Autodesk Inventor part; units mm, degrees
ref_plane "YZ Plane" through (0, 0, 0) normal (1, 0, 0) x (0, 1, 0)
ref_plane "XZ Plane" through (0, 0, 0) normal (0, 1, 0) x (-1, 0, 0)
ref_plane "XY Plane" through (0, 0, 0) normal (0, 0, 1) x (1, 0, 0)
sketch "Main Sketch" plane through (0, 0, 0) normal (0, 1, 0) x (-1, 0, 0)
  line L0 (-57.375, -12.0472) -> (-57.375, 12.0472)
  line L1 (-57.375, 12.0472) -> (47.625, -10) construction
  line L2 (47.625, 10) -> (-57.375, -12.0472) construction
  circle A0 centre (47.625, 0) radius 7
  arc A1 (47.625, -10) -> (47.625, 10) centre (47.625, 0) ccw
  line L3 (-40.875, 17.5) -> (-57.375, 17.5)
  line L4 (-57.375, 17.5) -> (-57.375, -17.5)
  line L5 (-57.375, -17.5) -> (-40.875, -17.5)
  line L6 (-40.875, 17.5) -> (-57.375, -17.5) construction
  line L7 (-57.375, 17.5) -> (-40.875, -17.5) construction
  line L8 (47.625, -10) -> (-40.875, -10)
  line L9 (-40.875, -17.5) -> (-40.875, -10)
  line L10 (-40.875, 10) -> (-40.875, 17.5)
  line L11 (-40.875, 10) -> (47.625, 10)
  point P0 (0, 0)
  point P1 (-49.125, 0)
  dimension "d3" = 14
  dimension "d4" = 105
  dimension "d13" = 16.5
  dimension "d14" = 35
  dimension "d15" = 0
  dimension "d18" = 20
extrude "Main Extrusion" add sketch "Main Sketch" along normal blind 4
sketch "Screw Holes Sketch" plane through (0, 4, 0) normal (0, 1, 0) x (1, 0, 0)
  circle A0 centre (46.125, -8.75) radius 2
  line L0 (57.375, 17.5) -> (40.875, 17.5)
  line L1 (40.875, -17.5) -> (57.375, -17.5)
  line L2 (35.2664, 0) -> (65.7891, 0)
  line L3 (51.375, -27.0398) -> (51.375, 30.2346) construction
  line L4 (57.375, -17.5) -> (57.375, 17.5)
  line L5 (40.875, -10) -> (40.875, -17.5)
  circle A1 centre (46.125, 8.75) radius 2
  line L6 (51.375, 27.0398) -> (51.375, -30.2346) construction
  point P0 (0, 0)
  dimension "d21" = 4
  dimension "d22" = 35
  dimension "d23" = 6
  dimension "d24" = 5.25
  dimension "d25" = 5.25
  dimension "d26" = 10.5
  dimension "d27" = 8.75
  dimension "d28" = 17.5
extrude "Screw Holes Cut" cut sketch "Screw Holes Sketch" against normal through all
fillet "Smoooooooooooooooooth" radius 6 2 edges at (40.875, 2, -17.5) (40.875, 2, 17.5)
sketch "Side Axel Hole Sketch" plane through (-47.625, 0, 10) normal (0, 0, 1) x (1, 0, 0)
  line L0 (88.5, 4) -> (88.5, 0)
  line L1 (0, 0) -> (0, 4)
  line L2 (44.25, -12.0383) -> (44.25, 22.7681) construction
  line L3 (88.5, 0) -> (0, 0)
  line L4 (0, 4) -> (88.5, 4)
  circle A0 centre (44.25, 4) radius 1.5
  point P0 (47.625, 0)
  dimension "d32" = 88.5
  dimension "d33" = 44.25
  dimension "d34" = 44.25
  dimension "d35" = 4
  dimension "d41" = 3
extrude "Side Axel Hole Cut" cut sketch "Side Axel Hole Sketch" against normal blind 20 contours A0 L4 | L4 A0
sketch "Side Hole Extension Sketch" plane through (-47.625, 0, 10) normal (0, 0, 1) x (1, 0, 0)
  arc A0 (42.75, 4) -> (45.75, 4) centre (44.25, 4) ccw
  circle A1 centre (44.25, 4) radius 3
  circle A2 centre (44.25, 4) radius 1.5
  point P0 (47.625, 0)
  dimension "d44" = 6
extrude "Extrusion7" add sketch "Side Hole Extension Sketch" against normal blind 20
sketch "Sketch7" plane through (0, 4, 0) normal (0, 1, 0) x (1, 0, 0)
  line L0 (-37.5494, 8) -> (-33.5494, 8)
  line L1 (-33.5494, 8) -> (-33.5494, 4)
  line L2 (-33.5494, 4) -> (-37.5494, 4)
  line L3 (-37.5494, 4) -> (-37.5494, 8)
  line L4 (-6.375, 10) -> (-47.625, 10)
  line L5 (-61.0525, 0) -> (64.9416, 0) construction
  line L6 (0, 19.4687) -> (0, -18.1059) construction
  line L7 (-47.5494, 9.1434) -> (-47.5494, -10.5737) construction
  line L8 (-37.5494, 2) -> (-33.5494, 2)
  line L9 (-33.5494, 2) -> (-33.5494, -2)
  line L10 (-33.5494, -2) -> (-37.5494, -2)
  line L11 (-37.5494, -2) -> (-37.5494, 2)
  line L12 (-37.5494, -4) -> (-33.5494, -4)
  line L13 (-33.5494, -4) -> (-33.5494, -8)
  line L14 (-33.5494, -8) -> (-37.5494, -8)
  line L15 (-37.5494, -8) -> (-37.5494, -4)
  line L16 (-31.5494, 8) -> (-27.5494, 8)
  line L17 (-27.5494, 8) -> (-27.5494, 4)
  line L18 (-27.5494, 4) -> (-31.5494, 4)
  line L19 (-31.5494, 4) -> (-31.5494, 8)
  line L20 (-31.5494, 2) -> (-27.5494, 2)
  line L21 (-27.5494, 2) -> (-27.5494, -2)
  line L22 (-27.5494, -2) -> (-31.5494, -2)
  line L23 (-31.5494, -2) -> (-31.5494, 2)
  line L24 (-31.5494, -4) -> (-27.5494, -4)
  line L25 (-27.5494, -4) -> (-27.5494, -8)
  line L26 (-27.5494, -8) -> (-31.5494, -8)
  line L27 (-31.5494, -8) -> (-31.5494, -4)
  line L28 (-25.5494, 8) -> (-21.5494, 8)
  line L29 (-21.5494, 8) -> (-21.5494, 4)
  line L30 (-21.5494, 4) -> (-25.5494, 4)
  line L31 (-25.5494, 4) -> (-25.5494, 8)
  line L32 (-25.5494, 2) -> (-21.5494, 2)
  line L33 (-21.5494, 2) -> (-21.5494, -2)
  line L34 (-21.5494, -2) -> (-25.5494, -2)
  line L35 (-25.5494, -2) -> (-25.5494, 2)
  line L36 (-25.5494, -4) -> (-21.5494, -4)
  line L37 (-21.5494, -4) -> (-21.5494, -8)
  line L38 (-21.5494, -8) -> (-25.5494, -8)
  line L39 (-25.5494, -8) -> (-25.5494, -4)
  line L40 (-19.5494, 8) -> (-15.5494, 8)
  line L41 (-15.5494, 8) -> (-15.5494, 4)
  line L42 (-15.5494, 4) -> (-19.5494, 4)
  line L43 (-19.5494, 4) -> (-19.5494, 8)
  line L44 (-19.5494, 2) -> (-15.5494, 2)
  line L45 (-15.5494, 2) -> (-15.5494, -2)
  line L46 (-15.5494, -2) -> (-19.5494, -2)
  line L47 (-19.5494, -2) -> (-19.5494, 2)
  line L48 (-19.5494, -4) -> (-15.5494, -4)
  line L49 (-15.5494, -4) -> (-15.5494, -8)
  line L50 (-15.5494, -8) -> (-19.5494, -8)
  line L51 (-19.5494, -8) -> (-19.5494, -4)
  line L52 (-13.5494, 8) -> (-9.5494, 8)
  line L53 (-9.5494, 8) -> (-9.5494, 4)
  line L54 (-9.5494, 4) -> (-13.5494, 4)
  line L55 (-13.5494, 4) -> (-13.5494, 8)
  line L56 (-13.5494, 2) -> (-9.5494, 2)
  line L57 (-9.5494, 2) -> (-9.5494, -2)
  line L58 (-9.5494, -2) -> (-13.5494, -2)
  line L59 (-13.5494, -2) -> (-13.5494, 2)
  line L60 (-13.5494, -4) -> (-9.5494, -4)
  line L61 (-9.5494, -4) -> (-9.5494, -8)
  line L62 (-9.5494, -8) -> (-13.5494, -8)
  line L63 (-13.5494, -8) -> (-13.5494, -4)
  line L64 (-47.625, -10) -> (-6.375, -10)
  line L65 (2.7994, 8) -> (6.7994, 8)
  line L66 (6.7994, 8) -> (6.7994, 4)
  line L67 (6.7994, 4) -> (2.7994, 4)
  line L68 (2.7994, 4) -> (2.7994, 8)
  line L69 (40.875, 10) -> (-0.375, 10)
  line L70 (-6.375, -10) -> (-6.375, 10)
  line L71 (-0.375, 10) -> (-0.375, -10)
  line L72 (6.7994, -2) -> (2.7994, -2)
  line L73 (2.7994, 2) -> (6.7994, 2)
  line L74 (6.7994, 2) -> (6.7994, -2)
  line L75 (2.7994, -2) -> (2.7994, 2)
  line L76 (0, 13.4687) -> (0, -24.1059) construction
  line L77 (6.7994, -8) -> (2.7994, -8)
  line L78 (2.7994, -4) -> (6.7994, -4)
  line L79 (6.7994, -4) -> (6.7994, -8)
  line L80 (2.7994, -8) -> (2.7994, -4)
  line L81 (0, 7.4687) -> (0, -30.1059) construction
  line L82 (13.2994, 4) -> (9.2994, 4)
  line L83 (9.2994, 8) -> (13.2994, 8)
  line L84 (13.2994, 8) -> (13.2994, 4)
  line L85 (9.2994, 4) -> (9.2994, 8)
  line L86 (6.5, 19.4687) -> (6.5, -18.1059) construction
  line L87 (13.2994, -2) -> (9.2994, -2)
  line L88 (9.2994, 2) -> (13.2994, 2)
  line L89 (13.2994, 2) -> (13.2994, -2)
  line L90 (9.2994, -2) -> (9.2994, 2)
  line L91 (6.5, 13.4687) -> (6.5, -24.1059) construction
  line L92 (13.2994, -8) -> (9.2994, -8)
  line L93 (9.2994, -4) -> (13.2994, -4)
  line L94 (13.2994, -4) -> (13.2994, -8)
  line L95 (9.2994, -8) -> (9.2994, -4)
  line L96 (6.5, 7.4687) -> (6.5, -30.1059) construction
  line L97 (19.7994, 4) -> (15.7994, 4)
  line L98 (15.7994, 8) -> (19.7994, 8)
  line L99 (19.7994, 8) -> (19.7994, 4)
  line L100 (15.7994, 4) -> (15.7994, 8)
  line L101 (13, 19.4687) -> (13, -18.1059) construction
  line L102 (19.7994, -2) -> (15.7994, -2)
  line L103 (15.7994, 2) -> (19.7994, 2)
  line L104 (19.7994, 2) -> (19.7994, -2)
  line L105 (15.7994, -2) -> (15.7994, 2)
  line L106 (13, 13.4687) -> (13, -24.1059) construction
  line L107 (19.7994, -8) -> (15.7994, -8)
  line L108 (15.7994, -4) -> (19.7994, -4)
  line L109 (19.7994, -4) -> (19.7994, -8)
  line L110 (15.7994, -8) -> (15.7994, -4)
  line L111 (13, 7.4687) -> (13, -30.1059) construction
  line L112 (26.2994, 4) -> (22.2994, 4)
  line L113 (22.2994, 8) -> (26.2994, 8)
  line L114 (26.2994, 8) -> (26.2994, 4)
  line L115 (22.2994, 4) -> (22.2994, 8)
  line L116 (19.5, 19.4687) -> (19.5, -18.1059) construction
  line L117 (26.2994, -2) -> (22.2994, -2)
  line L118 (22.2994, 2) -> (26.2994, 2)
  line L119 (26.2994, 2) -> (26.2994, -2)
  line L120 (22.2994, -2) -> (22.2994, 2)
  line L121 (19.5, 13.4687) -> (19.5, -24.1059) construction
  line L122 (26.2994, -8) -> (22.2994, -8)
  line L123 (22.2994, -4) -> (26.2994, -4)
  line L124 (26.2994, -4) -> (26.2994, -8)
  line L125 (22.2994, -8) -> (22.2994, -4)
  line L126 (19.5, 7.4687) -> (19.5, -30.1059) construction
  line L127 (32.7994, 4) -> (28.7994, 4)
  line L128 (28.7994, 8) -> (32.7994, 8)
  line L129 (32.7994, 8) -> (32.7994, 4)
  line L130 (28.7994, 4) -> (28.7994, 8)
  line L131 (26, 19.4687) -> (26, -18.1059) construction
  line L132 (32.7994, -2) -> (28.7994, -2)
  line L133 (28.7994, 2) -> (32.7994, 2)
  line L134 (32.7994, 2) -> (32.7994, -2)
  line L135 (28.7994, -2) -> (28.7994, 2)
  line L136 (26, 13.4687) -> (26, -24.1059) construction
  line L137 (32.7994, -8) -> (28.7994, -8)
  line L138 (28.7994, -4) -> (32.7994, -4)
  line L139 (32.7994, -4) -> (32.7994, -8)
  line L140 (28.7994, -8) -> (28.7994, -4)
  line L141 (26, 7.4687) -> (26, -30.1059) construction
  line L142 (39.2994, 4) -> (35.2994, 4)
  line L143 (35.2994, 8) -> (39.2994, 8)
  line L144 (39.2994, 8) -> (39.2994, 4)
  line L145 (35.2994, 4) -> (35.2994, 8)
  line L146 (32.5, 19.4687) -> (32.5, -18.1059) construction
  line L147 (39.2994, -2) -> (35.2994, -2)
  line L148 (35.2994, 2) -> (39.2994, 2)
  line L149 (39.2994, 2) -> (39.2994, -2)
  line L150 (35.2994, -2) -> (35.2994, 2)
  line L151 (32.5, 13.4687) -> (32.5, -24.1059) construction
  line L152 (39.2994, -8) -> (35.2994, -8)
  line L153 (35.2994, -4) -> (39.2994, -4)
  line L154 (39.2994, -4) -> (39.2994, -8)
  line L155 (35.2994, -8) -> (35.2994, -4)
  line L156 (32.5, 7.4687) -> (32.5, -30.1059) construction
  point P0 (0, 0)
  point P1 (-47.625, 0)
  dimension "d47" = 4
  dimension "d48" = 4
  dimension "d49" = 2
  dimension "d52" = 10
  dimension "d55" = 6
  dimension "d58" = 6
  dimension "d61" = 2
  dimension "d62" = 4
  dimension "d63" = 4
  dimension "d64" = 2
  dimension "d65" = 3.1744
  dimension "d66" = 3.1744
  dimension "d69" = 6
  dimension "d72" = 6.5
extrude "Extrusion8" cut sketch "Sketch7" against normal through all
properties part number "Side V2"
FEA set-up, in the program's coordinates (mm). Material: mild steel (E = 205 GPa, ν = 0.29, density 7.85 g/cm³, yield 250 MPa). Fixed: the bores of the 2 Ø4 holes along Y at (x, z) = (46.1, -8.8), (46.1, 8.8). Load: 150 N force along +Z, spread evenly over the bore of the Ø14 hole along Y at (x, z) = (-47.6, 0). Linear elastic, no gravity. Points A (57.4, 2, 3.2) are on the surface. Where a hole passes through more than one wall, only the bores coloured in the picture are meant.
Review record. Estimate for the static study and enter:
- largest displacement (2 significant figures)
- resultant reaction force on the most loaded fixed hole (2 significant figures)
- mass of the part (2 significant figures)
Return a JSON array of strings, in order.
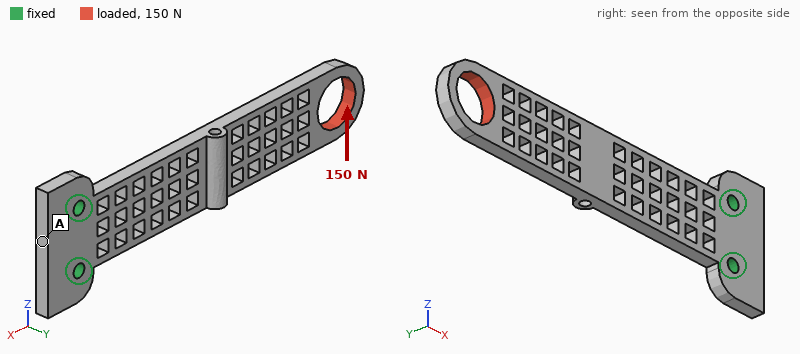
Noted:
["0.16 mm", "790 N", "57 g"]
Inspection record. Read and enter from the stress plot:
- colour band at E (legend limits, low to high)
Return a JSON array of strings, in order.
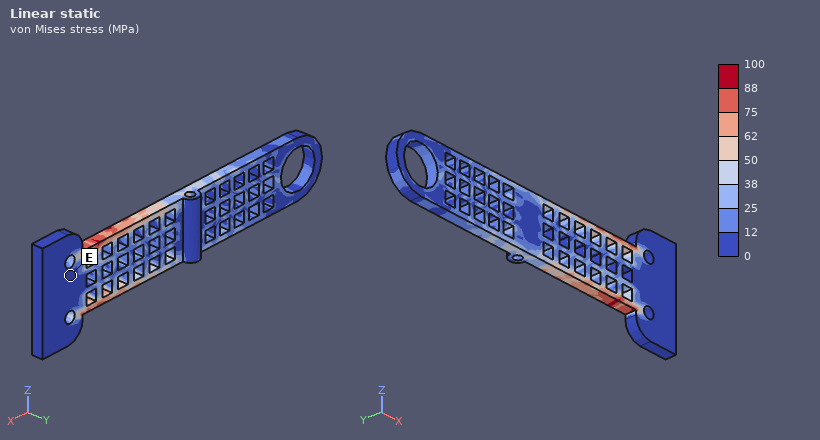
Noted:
["0 to 12 MPa"]
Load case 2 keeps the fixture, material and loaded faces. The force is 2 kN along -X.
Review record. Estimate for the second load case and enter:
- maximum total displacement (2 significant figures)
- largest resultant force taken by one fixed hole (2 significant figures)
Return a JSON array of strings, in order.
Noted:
["35 µm", "1.0 kN"]
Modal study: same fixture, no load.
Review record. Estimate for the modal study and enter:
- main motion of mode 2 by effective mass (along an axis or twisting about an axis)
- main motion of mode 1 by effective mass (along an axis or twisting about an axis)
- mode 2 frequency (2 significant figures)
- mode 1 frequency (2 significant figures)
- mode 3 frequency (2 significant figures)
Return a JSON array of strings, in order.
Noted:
["along Z", "along Y", "1500 Hz", "300 Hz", "1800 Hz"]
